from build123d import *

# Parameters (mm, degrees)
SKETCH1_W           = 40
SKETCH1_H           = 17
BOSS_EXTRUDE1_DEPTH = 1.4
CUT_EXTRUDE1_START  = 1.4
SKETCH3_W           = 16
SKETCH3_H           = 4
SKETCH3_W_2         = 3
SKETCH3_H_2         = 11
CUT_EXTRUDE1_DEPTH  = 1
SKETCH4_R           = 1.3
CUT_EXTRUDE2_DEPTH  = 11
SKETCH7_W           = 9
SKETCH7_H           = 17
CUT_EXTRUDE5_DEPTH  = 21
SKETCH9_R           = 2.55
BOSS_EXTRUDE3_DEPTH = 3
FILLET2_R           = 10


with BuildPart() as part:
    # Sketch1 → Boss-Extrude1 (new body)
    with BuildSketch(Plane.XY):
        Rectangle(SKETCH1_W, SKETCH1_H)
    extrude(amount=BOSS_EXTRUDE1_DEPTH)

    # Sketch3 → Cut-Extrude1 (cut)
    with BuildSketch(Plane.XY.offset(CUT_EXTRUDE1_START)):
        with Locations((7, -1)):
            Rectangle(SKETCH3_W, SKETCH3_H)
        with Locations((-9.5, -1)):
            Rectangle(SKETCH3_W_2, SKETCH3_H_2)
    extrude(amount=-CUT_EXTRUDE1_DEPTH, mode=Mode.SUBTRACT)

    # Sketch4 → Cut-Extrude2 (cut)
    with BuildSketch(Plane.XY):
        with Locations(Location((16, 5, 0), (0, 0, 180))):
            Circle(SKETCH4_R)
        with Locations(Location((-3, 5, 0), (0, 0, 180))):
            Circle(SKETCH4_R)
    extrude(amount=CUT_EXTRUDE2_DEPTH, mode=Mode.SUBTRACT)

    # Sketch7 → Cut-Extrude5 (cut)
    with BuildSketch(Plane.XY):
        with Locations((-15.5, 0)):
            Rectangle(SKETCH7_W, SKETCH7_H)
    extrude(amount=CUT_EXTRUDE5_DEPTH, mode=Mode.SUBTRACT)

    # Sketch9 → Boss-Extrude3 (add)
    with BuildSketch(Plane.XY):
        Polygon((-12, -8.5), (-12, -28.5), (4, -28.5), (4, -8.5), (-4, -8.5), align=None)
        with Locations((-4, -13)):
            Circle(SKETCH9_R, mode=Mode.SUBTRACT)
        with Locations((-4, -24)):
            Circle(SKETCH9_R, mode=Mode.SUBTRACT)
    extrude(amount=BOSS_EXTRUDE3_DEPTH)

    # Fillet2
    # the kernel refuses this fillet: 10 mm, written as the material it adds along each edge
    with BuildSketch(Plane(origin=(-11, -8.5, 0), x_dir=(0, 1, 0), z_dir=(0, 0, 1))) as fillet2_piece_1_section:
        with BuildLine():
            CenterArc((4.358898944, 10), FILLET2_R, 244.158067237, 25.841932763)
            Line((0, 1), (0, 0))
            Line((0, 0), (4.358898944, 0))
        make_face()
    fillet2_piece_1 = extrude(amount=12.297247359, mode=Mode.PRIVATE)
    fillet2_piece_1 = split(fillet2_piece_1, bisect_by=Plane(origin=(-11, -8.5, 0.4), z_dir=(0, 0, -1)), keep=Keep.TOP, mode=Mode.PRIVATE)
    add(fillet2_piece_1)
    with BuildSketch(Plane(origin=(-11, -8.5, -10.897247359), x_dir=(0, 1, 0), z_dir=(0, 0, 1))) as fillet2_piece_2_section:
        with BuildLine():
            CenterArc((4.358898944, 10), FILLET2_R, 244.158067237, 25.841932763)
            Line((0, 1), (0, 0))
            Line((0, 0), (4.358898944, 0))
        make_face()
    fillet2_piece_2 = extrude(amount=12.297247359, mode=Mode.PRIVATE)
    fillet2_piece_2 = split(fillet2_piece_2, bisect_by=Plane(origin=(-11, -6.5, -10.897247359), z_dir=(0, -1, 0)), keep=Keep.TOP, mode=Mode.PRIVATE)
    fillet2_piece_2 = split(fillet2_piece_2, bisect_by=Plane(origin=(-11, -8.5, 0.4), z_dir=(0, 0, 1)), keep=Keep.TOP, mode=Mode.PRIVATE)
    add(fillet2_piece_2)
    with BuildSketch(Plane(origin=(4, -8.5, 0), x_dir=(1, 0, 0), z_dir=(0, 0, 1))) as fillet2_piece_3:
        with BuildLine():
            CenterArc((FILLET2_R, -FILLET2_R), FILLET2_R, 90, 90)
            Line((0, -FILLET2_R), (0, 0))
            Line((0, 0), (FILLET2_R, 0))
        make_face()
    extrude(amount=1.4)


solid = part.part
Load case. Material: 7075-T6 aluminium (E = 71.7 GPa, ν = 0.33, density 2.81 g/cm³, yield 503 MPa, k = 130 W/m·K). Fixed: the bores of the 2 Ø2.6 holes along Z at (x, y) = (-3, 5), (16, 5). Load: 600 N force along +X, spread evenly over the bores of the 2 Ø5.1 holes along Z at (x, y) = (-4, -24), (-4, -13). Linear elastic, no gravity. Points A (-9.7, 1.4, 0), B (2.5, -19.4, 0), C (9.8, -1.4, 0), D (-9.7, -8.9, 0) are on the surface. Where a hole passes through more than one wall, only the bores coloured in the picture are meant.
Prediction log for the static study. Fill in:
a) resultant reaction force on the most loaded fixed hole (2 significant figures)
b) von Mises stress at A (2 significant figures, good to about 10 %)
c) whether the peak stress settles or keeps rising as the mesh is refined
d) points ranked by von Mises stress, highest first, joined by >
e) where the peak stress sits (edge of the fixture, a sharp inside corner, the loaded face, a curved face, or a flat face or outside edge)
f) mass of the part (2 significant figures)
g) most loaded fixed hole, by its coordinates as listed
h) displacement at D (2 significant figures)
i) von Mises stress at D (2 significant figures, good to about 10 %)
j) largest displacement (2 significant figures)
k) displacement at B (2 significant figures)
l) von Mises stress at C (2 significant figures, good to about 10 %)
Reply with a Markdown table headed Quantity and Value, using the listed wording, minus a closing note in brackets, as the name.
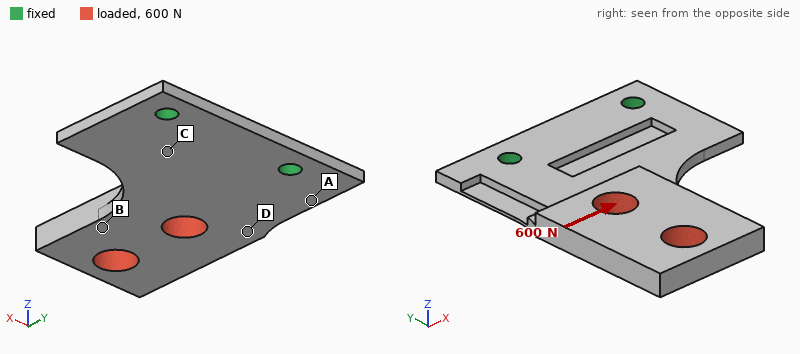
| Quantity | Value |
|---|---|
| resultant reaction force on the most loaded fixed hole | 770 N |
| von Mises stress at A | 93 MPa |
| whether the peak stress settles or keeps rising as the mesh is refined | keeps rising |
| points ranked by von Mises stress, highest first, joined by > | C > A > D > B |
| where the peak stress sits | edge of the fixture |
| mass of the part | 4.2 g |
| most loaded fixed hole, by its coordinates as listed | (16, 5) |
| displacement at D | 0.12 mm |
| von Mises stress at D | 36 MPa |
| largest displacement | 0.26 mm |
| displacement at B | 0.096 mm |
| von Mises stress at C | 140 MPa |
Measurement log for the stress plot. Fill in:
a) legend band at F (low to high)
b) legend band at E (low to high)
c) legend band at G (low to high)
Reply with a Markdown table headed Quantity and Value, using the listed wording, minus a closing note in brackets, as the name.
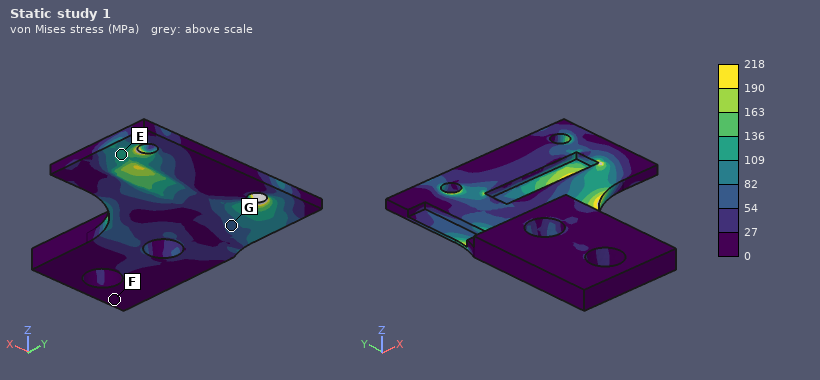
| Quantity | Value |
|---|---|
| legend band at F | 0 to 27 MPa |
| legend band at E | 109 to 136 MPa |
| legend band at G | 54 to 82 MPa |
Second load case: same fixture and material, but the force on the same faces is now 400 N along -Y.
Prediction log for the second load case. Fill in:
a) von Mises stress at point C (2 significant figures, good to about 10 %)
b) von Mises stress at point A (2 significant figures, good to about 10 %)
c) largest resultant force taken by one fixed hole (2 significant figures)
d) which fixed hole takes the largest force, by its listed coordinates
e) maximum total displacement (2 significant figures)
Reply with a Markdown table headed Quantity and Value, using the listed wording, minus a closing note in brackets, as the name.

| Quantity | Value |
|---|---|
| von Mises stress at point C | 44 MPa |
| von Mises stress at point A | 36 MPa |
| largest resultant force taken by one fixed hole | 410 N |
| which fixed hole takes the largest force, by its listed coordinates | (-3, 5) |
| maximum total displacement | 0.50 mm |
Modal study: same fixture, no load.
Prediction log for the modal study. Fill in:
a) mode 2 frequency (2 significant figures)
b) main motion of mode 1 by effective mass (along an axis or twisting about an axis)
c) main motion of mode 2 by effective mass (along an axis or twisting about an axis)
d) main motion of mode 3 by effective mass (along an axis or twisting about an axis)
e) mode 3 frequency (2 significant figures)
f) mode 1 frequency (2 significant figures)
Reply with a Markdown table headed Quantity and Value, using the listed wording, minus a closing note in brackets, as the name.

| Quantity | Value |
|---|---|
| mode 2 frequency | 3900 Hz |
| main motion of mode 1 by effective mass | along Z |
| main motion of mode 2 by effective mass | twisting about Y |
| main motion of mode 3 by effective mass | along Z |
| mode 3 frequency | 6800 Hz |
| mode 1 frequency | 790 Hz |
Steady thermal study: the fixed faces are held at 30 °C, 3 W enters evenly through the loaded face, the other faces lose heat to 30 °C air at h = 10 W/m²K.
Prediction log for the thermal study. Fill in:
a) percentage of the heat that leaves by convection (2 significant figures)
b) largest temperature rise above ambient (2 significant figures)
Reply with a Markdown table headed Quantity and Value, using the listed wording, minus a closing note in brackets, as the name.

| Quantity | Value |
|---|---|
| percentage of the heat that leaves by convection | 6.3 % |
| largest temperature rise above ambient | 20 K |
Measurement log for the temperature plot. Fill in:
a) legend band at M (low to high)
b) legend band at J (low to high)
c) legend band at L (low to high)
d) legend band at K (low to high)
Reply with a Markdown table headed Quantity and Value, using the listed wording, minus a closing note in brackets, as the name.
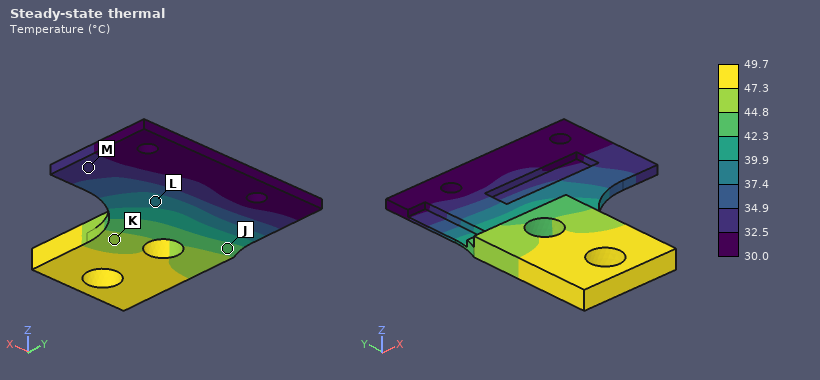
| Quantity | Value |
|---|---|
| legend band at M | 32.5 to 34.9 °C |
| legend band at J | 42.3 to 44.8 °C |
| legend band at L | 37.4 to 39.9 °C |
| legend band at K | 44.8 to 47.3 °C |
